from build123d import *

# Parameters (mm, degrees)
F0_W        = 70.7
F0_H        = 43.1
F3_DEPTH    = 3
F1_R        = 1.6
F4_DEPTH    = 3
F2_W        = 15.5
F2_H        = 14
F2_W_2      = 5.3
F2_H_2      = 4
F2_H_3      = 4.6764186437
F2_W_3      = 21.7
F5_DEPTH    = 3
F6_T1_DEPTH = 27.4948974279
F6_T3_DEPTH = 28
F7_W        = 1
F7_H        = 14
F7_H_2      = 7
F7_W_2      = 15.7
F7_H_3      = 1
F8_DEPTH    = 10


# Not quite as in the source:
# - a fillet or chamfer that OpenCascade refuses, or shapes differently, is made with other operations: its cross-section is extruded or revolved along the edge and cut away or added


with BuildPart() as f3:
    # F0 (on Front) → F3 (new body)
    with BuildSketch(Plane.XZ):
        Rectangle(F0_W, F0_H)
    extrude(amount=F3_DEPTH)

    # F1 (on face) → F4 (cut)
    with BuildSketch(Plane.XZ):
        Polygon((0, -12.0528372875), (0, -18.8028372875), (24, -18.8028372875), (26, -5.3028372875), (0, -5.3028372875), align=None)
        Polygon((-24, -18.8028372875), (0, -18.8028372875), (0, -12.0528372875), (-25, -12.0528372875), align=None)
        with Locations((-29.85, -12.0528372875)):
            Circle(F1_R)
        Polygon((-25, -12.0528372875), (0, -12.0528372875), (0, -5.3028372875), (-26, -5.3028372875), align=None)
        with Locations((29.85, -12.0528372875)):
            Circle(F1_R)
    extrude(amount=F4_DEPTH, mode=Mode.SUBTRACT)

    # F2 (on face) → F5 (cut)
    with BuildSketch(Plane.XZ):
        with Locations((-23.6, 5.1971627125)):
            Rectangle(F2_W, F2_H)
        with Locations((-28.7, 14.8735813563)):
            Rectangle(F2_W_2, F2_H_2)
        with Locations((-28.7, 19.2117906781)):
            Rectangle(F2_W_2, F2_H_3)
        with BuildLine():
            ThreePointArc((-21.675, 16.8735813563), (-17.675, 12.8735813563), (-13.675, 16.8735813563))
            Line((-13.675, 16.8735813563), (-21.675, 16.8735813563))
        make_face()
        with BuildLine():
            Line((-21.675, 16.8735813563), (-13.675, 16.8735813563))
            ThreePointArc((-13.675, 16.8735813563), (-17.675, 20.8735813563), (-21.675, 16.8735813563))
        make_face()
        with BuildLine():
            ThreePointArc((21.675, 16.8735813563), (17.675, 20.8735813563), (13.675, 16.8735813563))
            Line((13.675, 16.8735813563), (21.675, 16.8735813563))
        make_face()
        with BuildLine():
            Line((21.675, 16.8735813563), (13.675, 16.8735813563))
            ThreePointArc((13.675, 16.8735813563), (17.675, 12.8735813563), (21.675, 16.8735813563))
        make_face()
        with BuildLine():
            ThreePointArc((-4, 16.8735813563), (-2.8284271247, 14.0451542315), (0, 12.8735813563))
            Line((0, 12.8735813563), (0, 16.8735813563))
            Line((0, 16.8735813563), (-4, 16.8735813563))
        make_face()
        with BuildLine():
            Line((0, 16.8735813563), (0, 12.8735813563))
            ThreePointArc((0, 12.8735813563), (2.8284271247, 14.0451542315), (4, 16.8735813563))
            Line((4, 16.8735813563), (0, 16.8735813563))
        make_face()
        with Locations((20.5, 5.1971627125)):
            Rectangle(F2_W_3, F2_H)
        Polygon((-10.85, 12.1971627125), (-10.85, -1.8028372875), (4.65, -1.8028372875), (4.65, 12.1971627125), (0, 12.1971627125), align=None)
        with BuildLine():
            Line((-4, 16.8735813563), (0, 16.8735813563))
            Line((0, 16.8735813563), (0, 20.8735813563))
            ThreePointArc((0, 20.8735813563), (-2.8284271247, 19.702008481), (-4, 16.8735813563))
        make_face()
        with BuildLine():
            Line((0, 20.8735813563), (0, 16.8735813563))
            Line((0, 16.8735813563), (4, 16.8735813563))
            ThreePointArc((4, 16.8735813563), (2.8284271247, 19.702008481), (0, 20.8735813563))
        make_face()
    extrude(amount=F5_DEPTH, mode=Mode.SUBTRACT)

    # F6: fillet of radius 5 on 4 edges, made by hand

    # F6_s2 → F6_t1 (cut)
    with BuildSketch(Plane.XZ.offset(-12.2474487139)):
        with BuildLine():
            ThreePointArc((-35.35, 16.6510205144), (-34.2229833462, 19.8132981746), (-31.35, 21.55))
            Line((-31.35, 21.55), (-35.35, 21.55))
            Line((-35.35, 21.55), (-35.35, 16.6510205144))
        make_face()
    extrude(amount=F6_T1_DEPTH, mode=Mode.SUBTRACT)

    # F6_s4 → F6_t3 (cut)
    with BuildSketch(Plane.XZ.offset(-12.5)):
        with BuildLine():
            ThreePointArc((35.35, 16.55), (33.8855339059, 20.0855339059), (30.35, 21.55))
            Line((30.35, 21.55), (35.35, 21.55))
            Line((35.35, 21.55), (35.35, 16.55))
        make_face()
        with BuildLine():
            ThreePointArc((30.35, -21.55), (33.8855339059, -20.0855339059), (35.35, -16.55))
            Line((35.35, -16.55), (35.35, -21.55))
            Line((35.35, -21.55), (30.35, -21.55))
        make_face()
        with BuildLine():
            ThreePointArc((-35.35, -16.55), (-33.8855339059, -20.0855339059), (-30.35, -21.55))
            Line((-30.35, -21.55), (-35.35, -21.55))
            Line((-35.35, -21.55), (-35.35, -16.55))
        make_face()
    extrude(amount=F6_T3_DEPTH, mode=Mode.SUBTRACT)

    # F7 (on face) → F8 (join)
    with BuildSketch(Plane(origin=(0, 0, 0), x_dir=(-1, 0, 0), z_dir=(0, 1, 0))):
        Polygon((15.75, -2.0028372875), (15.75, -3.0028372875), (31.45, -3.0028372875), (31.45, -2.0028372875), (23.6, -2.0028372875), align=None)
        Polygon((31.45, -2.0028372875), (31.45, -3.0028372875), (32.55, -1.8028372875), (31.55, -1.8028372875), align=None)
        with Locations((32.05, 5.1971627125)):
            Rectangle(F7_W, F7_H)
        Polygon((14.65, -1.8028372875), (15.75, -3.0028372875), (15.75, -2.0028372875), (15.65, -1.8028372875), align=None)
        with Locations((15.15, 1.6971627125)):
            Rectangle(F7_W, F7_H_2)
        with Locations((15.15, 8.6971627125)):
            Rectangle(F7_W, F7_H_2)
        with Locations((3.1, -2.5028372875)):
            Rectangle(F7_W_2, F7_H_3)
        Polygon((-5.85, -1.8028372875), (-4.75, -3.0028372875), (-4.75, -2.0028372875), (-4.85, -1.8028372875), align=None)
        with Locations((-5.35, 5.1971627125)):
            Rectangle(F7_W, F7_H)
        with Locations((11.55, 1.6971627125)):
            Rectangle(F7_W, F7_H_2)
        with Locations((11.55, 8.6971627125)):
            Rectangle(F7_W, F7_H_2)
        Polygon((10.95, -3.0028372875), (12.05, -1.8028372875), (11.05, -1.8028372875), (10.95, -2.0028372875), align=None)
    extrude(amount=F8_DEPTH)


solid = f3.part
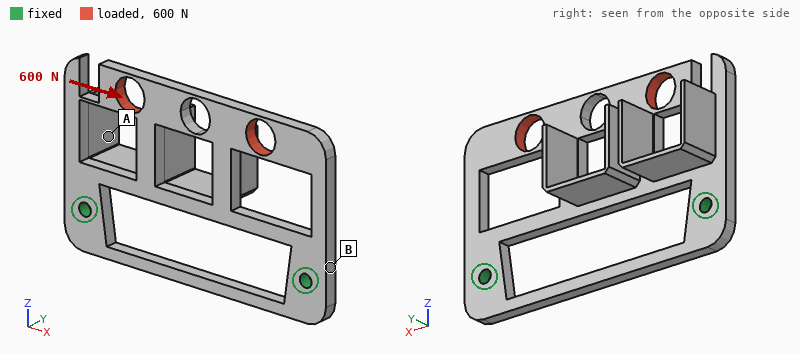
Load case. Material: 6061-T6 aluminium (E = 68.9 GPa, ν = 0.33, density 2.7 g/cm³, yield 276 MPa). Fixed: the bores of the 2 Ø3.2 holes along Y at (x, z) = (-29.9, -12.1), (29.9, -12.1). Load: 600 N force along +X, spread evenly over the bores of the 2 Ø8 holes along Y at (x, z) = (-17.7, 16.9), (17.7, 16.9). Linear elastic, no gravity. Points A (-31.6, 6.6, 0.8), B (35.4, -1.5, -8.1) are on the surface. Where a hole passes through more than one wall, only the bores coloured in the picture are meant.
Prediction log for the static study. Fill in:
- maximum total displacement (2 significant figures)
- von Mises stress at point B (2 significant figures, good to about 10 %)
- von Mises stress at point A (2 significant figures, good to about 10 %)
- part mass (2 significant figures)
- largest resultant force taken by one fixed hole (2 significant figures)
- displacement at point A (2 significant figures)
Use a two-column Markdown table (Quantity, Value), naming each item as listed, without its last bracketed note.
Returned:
| Quantity | Value |
|---|---|
| maximum total displacement | 0.17 mm |
| von Mises stress at point B | 52 MPa |
| von Mises stress at point A | 19 MPa |
| part mass | 14 g |
| largest resultant force taken by one fixed hole | 380 N |
| displacement at point A | 0.027 mm |
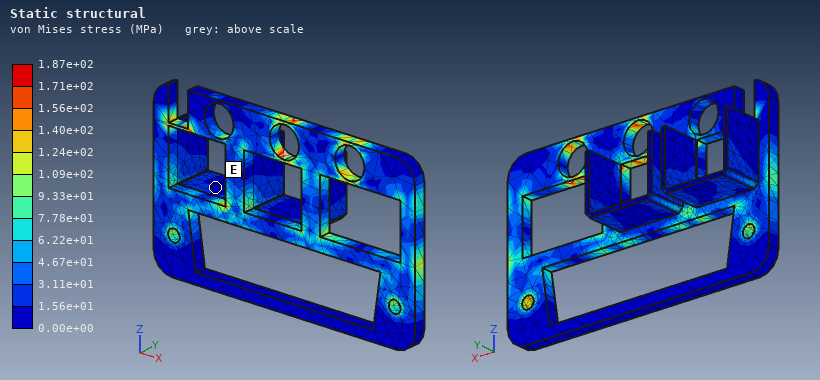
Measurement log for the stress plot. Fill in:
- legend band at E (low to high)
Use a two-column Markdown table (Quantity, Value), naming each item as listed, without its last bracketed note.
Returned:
| Quantity | Value |
|---|---|
| legend band at E | 0.00e+00 to 1.56e+01 MPa |
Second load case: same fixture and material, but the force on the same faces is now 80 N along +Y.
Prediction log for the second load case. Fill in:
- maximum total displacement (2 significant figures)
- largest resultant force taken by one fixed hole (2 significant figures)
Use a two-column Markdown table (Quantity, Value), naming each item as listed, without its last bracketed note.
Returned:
| Quantity | Value |
|---|---|
| maximum total displacement | 0.44 mm |
| largest resultant force taken by one fixed hole | 41 N |
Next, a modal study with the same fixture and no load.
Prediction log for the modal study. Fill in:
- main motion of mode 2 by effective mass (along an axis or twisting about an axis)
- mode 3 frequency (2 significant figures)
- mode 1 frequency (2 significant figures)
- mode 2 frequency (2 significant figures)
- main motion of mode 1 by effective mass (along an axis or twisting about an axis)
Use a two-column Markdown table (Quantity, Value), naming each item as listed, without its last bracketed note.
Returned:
| Quantity | Value |
|---|---|
| main motion of mode 2 by effective mass | twisting about Z |
| mode 3 frequency | 3300 Hz |
| mode 1 frequency | 1200 Hz |
| mode 2 frequency | 2500 Hz |
| main motion of mode 1 by effective mass | along Y |
